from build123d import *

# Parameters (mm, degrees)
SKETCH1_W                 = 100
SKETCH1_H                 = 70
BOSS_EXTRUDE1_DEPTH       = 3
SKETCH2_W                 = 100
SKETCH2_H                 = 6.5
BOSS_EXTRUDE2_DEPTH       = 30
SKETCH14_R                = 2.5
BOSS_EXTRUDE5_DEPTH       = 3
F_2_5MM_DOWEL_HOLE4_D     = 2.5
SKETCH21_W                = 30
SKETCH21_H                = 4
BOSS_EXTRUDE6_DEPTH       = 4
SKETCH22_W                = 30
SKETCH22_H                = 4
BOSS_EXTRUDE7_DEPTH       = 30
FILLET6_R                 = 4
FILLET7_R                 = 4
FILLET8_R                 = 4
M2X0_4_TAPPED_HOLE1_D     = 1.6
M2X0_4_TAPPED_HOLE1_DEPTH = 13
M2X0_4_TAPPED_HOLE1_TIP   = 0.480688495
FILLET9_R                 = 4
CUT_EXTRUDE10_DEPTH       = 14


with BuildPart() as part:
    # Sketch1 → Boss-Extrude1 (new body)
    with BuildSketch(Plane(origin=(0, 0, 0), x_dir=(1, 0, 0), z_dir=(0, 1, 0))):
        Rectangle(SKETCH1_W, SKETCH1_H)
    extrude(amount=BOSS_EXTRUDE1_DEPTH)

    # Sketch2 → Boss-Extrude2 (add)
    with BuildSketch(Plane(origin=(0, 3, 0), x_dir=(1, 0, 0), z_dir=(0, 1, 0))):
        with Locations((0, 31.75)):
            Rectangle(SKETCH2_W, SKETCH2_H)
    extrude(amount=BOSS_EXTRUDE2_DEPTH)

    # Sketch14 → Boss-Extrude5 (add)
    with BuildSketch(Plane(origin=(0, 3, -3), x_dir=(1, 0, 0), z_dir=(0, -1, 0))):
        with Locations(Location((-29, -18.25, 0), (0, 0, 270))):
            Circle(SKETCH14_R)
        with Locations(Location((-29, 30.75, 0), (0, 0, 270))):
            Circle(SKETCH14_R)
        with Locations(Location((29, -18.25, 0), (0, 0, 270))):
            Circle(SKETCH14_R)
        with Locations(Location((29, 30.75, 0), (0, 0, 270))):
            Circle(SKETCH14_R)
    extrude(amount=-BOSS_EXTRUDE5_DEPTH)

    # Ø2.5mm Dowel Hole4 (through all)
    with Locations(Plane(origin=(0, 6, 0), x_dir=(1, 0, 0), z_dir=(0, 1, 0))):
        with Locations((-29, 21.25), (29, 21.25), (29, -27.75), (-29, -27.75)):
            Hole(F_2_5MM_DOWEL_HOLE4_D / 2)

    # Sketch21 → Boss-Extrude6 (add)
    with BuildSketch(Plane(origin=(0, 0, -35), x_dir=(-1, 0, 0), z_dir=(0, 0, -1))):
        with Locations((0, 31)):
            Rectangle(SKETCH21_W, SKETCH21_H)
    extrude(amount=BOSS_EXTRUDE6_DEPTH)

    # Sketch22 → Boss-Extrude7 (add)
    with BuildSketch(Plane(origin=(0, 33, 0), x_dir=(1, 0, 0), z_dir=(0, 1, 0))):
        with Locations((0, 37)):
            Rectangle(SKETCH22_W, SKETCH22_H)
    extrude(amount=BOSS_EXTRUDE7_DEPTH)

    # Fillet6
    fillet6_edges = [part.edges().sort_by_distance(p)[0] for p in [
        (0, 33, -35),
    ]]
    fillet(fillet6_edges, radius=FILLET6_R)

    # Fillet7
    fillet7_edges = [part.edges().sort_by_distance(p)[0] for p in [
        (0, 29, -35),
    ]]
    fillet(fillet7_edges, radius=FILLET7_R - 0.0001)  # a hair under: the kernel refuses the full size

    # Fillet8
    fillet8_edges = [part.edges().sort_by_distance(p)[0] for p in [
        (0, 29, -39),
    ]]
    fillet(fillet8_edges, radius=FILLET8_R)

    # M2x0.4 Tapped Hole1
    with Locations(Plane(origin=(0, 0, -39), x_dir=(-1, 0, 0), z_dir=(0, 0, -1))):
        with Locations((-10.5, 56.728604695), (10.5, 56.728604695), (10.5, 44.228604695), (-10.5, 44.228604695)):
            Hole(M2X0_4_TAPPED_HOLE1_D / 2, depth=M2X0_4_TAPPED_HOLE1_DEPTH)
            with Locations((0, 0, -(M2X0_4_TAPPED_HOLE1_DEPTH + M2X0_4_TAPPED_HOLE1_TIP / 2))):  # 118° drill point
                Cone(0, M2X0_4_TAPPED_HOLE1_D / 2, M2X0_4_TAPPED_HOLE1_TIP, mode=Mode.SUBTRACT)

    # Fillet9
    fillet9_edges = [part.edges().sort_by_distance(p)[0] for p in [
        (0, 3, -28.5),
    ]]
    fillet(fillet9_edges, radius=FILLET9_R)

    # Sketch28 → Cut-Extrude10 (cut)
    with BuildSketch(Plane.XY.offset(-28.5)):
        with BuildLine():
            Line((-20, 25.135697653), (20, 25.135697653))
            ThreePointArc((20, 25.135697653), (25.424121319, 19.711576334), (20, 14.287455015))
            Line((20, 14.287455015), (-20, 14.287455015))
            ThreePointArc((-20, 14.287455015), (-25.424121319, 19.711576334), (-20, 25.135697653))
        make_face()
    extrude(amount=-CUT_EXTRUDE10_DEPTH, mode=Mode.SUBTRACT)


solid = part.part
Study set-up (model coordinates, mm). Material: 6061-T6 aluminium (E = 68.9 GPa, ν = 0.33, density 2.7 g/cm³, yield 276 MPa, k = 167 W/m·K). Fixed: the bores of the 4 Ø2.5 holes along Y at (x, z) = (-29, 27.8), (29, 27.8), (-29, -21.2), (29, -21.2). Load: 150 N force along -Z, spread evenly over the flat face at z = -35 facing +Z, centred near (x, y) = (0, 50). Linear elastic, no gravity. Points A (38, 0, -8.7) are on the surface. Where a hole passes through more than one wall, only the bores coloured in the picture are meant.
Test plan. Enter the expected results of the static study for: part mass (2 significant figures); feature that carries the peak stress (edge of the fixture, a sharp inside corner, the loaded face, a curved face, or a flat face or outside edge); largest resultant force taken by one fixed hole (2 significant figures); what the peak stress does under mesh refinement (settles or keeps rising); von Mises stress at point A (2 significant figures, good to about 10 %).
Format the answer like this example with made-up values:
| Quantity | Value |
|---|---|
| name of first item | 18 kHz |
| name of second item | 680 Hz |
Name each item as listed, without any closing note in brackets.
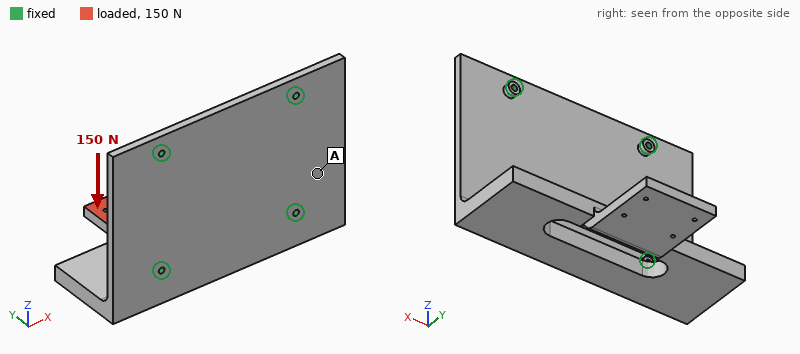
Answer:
| Quantity | Value |
|---|---|
| part mass | 110 g |
| feature that carries the peak stress | edge of the fixture |
| largest resultant force taken by one fixed hole | 94 N |
| what the peak stress does under mesh refinement | keeps rising |
| von Mises stress at point A | 8.4 MPa |
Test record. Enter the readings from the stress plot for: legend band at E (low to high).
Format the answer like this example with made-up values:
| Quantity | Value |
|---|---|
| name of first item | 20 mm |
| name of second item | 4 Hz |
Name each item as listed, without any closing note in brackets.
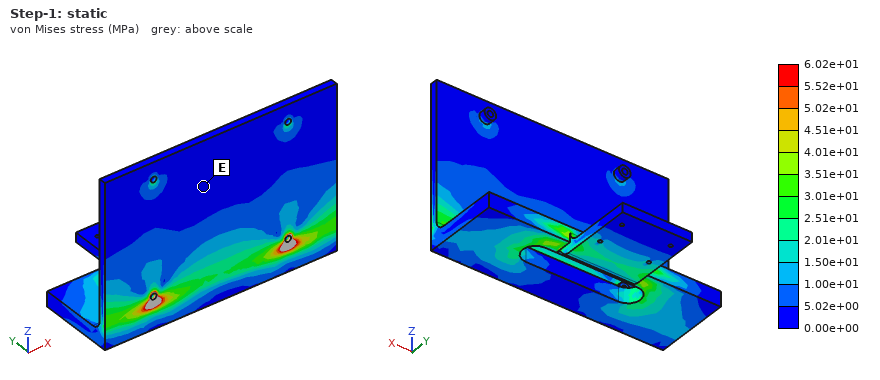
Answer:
| Quantity | Value |
|---|---|
| legend band at E | 0.00e+00 to 5.02e+00 MPa |
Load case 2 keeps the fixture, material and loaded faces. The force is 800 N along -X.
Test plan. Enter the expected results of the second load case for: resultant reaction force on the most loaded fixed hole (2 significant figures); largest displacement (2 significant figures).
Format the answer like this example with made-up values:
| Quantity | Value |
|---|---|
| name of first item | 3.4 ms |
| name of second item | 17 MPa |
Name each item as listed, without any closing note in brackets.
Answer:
| Quantity | Value |
|---|---|
| resultant reaction force on the most loaded fixed hole | 770 N |
| largest displacement | 0.12 mm |
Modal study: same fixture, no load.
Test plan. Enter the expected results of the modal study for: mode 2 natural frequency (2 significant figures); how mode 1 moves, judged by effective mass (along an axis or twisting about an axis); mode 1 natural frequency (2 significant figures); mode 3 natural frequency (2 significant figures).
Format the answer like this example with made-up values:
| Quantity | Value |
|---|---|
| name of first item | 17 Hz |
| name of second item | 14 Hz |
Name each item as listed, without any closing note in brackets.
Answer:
| Quantity | Value |
|---|---|
| mode 2 natural frequency | 2600 Hz |
| how mode 1 moves, judged by effective mass | along Z |
| mode 1 natural frequency | 850 Hz |
| mode 3 natural frequency | 2900 Hz |
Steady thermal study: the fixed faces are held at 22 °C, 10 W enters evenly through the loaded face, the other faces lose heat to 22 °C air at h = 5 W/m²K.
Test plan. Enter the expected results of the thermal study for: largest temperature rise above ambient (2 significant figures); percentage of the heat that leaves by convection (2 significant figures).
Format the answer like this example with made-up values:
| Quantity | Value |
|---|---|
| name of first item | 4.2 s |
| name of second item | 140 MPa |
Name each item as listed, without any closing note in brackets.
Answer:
| Quantity | Value |
|---|---|
| largest temperature rise above ambient | 27 K |
| percentage of the heat that leaves by convection | 5.3 % |
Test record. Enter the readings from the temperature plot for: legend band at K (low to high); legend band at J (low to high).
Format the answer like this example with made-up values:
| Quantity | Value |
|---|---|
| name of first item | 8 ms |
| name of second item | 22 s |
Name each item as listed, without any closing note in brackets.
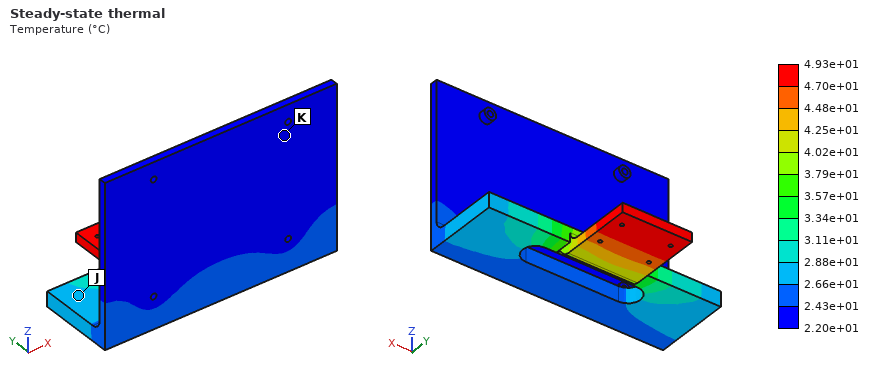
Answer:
| Quantity | Value |
|---|---|
| legend band at K | 2.20e+01 to 2.43e+01 °C |
| legend band at J | 2.66e+01 to 2.88e+01 °C |
